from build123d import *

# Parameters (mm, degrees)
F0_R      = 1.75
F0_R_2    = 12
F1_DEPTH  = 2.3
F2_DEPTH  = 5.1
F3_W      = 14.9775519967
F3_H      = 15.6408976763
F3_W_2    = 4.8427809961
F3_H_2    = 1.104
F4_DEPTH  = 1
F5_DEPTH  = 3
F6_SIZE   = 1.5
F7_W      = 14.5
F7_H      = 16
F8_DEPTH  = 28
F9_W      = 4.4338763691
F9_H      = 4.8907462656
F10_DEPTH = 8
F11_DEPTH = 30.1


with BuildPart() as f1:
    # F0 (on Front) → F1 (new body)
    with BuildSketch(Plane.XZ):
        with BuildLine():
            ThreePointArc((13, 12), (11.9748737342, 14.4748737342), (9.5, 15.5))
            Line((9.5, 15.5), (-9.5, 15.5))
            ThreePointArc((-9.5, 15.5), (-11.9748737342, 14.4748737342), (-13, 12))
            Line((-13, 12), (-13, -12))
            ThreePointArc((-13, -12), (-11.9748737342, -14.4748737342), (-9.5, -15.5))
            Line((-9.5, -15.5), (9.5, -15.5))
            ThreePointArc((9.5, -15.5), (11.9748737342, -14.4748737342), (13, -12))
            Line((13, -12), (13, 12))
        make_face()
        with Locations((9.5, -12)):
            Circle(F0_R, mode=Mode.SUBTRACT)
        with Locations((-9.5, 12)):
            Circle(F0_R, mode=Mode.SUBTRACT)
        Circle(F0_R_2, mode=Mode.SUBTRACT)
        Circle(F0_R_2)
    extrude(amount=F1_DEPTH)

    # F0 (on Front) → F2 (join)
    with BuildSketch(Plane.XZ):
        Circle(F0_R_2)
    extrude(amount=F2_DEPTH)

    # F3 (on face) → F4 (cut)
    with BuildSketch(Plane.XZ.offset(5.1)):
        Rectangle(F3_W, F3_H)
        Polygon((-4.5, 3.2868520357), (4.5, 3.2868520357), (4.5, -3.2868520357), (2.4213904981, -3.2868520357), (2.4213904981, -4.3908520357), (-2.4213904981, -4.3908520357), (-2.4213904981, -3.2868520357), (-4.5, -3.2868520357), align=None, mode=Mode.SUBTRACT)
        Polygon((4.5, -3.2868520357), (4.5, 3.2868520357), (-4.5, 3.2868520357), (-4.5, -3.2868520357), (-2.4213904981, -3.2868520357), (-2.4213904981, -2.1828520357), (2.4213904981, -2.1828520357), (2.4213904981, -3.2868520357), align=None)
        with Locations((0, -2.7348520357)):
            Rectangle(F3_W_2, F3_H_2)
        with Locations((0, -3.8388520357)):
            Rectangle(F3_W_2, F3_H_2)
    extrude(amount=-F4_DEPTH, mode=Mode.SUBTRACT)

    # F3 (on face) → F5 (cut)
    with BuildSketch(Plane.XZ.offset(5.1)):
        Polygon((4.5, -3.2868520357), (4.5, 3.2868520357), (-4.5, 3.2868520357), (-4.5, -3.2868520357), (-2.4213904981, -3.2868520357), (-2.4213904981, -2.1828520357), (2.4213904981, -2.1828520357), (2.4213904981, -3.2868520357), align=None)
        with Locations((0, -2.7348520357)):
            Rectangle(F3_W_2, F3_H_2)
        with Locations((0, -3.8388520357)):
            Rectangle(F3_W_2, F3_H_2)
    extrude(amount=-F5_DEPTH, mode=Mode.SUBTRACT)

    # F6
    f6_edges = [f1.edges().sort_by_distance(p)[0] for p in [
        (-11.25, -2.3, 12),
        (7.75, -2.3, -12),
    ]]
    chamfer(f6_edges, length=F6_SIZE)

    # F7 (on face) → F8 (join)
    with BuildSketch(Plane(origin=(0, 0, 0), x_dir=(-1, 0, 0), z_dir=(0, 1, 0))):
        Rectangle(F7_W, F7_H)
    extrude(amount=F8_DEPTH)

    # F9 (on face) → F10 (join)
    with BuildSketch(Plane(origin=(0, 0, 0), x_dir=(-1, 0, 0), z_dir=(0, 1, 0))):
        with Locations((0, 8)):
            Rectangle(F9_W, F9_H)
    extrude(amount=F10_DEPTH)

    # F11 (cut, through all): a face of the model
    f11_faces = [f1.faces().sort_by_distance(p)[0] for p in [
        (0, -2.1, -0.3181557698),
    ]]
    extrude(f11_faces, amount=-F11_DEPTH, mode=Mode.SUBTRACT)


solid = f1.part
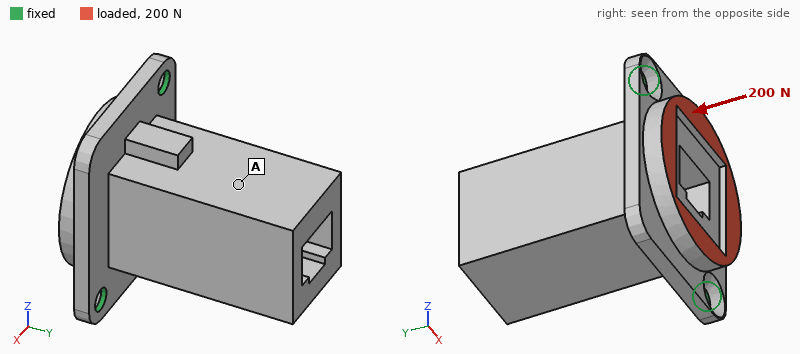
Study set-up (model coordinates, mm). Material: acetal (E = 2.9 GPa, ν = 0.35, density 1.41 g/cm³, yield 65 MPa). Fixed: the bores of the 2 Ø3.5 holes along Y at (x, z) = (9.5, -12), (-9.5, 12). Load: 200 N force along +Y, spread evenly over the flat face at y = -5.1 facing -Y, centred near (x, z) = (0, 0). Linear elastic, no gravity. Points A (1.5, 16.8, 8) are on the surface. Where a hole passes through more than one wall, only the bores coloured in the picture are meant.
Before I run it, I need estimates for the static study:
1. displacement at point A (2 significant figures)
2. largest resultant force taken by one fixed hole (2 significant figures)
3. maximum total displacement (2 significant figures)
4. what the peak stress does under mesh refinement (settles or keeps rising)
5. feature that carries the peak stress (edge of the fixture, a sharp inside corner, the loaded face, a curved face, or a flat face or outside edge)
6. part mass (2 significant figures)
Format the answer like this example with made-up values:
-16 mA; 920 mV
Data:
0.083 mm; 110 N; 0.13 mm; keeps rising; edge of the fixture; 10 g
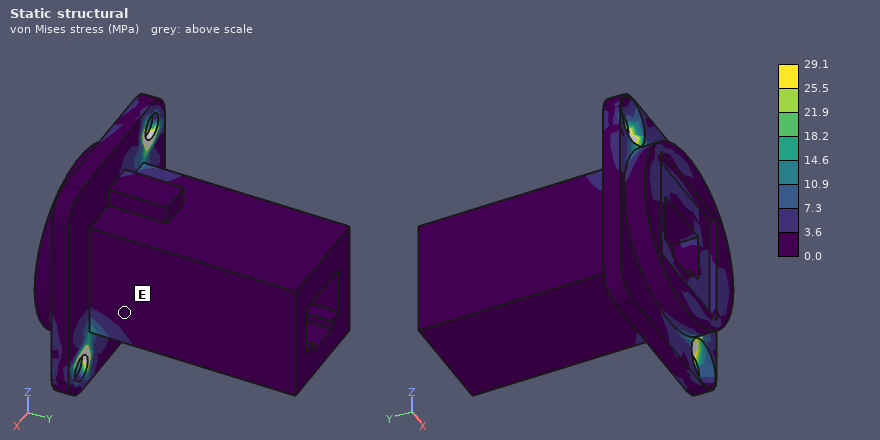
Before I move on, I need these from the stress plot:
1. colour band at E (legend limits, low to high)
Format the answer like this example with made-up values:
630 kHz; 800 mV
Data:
0.0 to 3.6 MPa
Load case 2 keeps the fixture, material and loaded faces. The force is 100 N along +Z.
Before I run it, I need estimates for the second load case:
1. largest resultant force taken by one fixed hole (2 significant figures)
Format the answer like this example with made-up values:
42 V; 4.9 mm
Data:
52 N
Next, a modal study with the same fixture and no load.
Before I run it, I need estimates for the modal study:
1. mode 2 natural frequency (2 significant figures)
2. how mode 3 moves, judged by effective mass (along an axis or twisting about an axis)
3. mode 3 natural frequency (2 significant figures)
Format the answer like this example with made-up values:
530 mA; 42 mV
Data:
1800 Hz; along Y; 2300 Hz
